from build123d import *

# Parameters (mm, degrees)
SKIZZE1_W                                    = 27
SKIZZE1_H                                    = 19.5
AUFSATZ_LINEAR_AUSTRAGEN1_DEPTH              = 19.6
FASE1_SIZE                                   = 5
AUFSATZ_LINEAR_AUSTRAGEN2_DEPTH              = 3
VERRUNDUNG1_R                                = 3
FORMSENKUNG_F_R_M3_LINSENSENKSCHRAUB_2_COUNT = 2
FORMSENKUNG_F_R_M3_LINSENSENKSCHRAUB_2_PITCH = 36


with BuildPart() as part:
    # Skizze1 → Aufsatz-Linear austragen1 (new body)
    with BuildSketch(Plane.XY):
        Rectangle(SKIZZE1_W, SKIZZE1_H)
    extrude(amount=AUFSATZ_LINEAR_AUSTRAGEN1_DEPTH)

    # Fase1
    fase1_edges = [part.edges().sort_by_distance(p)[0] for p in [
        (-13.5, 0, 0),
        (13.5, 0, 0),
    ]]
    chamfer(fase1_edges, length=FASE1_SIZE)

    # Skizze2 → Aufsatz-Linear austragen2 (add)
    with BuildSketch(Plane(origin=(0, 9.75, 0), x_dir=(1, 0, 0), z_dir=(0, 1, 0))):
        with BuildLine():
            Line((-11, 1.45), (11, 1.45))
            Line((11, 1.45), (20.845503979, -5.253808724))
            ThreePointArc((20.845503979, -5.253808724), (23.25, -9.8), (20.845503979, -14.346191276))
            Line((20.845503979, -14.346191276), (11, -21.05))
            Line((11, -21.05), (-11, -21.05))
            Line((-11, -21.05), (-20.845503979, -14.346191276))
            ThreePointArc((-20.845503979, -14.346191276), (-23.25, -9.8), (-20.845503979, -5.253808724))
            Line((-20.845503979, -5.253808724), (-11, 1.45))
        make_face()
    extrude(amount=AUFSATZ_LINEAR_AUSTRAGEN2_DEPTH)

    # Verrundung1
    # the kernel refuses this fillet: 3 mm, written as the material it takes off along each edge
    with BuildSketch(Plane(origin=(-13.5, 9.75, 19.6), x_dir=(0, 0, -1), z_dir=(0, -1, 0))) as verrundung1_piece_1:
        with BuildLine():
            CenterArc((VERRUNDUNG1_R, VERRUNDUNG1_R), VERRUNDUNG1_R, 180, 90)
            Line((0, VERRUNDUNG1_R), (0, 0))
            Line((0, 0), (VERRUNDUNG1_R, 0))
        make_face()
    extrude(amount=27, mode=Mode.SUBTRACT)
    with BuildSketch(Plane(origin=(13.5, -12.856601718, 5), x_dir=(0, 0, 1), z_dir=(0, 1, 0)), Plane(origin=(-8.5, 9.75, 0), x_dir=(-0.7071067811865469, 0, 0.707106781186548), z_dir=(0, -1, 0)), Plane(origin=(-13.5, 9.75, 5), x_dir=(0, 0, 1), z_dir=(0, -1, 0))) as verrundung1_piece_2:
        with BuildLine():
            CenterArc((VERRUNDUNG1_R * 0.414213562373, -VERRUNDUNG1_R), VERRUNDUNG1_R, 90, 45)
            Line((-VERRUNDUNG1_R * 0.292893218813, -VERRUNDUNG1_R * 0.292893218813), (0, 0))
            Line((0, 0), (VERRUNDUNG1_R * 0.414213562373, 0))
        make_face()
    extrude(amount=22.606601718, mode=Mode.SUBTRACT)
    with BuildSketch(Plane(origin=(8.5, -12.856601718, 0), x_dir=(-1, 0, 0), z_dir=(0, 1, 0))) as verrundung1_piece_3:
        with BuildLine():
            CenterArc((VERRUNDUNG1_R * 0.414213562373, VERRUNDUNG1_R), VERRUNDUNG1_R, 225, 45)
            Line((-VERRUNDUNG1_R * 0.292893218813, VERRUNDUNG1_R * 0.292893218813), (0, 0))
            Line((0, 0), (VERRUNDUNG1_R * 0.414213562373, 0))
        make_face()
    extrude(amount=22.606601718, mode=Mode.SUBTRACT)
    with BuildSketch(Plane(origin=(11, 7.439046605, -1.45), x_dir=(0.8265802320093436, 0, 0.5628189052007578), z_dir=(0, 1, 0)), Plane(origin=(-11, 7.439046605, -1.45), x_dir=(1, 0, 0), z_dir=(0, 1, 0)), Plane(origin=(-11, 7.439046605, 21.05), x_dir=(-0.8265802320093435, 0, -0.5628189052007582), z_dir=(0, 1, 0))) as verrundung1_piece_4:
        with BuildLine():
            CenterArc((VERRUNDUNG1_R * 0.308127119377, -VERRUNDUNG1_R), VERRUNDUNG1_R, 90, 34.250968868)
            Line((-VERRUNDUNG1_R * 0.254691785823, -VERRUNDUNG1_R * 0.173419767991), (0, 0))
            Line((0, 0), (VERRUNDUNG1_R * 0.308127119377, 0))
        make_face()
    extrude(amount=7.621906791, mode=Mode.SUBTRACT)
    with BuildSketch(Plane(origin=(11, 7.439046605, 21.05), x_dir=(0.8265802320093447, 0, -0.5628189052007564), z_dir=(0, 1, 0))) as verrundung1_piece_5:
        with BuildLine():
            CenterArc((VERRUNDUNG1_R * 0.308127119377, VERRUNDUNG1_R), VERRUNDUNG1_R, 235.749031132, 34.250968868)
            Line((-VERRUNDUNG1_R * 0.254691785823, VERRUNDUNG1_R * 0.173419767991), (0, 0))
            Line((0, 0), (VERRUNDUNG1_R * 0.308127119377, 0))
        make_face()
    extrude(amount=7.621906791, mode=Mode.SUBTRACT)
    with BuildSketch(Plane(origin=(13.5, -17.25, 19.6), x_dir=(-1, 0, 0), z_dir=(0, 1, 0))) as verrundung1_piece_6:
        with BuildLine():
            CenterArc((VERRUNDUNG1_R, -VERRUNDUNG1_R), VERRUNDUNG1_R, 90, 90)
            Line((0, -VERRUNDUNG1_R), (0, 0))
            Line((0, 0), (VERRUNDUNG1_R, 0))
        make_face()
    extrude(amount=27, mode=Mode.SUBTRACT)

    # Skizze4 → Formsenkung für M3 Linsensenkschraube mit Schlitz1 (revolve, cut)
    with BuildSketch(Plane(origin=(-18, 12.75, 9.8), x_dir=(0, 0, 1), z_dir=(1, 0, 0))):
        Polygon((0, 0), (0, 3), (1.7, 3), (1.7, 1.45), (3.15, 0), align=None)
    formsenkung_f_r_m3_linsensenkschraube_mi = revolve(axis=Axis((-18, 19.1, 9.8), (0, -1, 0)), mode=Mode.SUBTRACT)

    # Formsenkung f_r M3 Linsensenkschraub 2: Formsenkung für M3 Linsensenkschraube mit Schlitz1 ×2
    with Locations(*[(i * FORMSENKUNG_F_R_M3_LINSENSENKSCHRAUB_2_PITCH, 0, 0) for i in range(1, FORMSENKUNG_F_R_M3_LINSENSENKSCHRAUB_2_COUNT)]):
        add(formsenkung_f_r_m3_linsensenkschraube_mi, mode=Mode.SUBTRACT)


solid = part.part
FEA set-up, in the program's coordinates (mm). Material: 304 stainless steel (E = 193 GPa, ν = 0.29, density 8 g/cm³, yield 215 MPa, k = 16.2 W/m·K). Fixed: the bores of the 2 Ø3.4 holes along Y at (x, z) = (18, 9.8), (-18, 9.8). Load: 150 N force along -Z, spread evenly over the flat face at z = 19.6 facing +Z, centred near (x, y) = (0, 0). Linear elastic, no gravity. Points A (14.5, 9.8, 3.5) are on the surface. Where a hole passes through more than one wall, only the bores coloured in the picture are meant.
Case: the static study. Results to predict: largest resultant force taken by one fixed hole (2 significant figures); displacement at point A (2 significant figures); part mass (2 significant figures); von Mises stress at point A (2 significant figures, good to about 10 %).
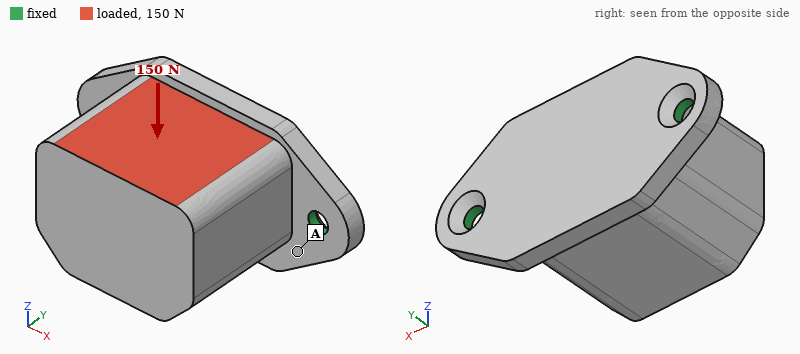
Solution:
75 N
3.6 µm
97 g
11 MPa
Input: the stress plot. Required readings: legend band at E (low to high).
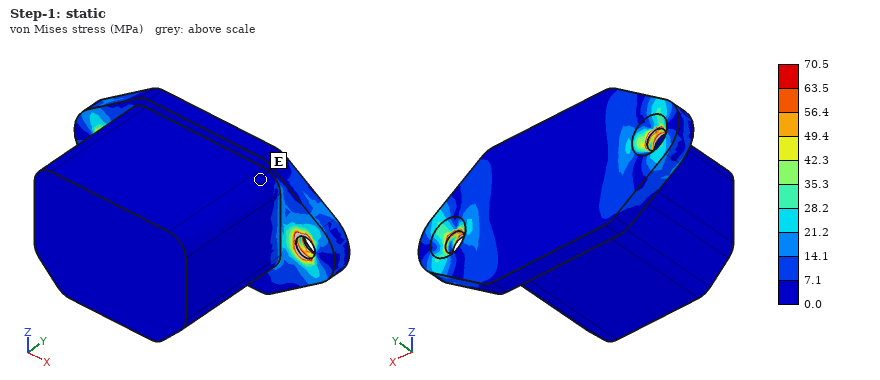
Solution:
0.0 to 7.1 MPa
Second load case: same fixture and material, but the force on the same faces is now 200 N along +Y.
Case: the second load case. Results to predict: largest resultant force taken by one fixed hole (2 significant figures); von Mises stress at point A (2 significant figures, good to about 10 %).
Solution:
100 N
11 MPa
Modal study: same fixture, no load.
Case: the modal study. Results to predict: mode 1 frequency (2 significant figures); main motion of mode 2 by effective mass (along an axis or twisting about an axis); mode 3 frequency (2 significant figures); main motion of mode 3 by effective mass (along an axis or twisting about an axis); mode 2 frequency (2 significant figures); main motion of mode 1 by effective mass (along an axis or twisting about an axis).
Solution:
2100 Hz
along Y
8700 Hz
along X
8000 Hz
along Z
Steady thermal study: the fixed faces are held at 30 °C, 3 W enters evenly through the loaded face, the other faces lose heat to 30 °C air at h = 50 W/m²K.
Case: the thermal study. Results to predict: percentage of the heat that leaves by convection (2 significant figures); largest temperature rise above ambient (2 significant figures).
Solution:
49 %
15 K
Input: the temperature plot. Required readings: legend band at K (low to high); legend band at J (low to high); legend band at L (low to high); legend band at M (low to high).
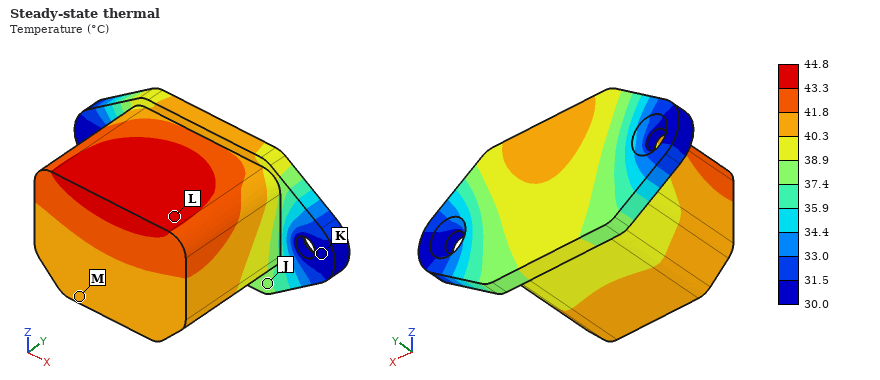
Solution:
30.0 to 31.5 °C
37.4 to 38.9 °C
43.3 to 44.8 °C
40.3 to 41.8 °C
